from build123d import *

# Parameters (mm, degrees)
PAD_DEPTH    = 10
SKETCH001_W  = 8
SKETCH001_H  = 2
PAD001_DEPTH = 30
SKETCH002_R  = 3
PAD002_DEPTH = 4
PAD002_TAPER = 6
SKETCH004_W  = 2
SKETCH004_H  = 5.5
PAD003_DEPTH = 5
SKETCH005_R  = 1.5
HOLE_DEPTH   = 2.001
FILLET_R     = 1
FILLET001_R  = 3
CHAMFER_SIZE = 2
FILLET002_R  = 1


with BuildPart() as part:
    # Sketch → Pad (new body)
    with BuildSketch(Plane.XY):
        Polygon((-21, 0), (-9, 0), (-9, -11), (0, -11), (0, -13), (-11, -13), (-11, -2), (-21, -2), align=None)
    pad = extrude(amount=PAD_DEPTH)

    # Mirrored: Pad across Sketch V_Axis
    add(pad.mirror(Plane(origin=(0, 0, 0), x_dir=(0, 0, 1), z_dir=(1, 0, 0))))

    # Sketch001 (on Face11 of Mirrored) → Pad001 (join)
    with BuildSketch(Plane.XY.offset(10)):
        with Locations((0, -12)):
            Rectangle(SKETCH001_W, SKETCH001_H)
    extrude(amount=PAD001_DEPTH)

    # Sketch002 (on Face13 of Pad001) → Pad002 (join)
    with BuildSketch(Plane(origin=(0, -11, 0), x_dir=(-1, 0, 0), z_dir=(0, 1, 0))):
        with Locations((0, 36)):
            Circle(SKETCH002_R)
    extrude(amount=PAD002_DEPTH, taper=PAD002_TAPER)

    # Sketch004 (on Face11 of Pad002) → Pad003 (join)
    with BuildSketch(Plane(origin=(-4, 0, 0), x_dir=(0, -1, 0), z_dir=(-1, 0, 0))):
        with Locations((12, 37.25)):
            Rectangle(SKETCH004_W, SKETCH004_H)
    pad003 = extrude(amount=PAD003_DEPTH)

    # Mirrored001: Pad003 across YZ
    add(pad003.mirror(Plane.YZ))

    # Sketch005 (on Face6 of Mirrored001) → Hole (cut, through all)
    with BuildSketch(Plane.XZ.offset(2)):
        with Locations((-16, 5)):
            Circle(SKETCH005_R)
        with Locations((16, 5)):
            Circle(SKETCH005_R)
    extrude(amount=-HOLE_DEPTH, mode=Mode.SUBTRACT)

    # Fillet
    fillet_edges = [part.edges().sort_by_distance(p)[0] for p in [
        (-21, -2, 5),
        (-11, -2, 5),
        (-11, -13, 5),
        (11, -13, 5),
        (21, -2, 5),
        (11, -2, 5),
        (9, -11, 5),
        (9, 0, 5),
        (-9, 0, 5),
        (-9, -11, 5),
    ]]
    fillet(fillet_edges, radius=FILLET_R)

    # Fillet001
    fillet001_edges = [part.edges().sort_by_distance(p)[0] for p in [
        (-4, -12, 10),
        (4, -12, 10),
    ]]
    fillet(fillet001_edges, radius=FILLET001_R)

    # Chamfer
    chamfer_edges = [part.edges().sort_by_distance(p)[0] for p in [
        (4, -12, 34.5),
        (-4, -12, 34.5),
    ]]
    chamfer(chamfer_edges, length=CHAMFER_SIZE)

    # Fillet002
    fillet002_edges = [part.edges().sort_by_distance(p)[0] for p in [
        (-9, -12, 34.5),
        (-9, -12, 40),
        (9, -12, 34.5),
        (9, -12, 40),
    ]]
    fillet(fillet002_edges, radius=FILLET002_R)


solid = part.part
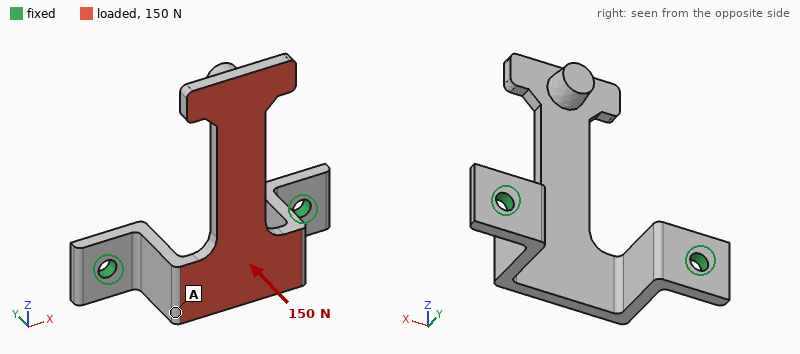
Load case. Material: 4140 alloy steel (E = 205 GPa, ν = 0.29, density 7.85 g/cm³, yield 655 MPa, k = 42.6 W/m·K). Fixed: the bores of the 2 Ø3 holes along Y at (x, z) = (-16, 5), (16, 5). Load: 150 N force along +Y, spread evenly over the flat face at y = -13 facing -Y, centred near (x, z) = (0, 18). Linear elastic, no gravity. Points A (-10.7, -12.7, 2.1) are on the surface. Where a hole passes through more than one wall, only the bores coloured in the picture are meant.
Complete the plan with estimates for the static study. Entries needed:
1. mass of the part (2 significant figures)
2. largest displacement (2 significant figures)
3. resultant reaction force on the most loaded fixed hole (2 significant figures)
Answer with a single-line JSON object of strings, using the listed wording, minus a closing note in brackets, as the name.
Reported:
{"mass of the part": "15 g", "largest displacement": "0.58 mm", "resultant reaction force on the most loaded fixed hole": "91 N"}
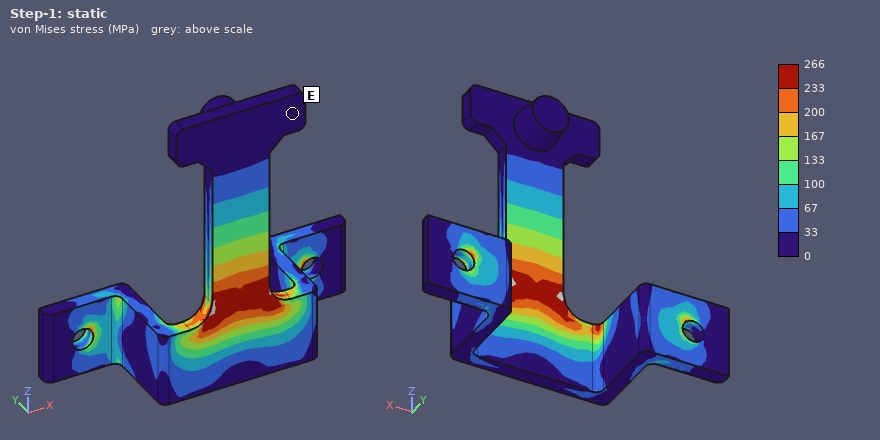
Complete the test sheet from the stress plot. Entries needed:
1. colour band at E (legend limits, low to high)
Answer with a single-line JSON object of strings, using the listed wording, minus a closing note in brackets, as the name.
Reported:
{"colour band at E": "0 to 33 MPa"}
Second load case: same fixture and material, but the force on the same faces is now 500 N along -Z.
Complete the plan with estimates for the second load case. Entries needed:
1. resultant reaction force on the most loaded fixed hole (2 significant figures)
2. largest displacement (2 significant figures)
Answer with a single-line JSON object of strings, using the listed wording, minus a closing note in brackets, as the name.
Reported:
{"resultant reaction force on the most loaded fixed hole": "250 N", "largest displacement": "0.32 mm"}
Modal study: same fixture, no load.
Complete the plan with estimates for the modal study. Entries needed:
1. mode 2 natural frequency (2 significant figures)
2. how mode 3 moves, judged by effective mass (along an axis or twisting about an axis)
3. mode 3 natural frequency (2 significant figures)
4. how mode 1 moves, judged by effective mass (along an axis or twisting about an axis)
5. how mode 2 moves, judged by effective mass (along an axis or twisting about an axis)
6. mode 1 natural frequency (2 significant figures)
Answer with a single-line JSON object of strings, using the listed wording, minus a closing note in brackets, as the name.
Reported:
{"mode 2 natural frequency": "2500 Hz", "how mode 3 moves, judged by effective mass": "along Z", "mode 3 natural frequency": "4500 Hz", "how mode 1 moves, judged by effective mass": "along Y", "how mode 2 moves, judged by effective mass": "along X", "mode 1 natural frequency": "940 Hz"}
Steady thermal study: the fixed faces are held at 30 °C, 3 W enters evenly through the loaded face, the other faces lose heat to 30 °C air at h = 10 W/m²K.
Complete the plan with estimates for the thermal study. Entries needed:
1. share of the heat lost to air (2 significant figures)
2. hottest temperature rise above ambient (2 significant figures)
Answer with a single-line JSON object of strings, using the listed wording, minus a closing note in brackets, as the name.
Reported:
{"share of the heat lost to air": "16 %", "hottest temperature rise above ambient": "69 K"}
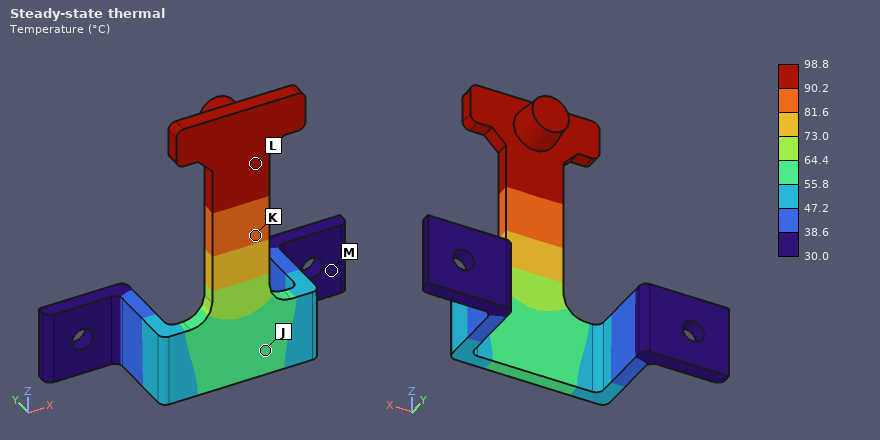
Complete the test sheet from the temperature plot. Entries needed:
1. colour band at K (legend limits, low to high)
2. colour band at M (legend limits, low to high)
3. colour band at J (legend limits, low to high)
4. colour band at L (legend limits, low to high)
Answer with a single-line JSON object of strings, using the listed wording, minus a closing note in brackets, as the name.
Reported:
{"colour band at K": "81.6 to 90.2 °C", "colour band at M": "30.0 to 38.6 °C", "colour band at J": "55.8 to 64.4 °C", "colour band at L": "90.2 to 98.8 °C"}
